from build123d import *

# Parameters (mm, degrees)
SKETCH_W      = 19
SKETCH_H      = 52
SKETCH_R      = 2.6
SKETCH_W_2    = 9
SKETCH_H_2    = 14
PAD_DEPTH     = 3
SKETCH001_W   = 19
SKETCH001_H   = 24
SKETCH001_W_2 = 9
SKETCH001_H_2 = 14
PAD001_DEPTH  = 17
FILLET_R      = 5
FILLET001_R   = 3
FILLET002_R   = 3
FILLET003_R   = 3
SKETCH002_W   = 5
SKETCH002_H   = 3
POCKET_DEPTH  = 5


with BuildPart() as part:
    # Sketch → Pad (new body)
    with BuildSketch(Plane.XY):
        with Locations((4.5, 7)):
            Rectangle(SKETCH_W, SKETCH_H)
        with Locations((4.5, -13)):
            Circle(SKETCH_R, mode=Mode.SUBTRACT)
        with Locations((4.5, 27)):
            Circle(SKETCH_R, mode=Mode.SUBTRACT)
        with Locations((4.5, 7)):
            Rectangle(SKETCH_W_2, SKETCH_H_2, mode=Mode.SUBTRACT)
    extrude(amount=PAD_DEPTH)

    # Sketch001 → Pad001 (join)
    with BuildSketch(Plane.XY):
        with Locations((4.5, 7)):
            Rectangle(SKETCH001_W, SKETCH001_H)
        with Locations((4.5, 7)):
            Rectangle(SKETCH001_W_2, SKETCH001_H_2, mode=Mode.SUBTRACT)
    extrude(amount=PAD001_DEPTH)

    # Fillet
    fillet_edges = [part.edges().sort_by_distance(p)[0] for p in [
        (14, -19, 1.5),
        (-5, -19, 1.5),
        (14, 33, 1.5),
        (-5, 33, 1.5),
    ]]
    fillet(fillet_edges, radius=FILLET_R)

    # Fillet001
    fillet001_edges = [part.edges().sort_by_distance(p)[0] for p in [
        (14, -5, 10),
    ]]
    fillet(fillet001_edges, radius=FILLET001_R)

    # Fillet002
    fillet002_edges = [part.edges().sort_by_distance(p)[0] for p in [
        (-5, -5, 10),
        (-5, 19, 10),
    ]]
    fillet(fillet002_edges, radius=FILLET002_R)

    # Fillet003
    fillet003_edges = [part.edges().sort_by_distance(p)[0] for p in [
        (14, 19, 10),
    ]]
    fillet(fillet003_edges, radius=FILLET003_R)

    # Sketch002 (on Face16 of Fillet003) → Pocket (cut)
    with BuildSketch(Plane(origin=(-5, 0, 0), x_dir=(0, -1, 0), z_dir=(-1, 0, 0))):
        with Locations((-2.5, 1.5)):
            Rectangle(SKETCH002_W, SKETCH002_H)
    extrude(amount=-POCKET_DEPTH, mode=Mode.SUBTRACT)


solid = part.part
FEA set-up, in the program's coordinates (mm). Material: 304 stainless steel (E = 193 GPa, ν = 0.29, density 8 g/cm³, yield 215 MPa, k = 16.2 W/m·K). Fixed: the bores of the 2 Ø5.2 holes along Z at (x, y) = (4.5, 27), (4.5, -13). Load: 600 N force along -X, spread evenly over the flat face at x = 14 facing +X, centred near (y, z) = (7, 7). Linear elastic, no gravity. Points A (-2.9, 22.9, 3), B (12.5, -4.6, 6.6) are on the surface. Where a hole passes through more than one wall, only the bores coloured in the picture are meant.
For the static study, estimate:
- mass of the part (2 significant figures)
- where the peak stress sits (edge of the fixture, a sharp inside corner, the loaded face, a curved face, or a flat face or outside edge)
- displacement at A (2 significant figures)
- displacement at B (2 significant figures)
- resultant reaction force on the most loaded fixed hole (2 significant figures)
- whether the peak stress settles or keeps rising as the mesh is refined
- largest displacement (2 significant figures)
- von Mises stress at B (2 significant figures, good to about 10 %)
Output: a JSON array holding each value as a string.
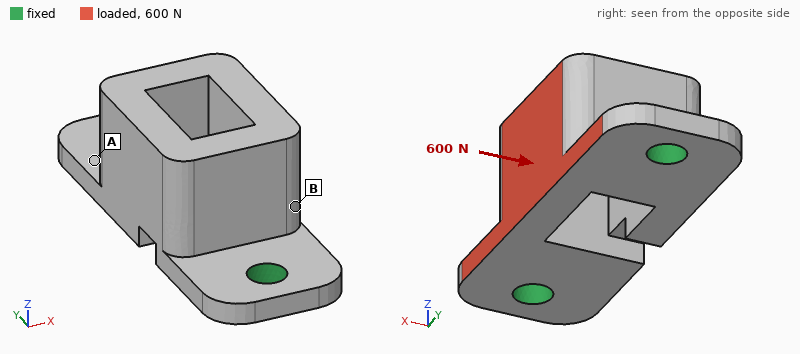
["55 g", "edge of the fixture", "3.4 µm", "7.9 µm", "310 N", "keeps rising", "16 µm", "7.1 MPa"]
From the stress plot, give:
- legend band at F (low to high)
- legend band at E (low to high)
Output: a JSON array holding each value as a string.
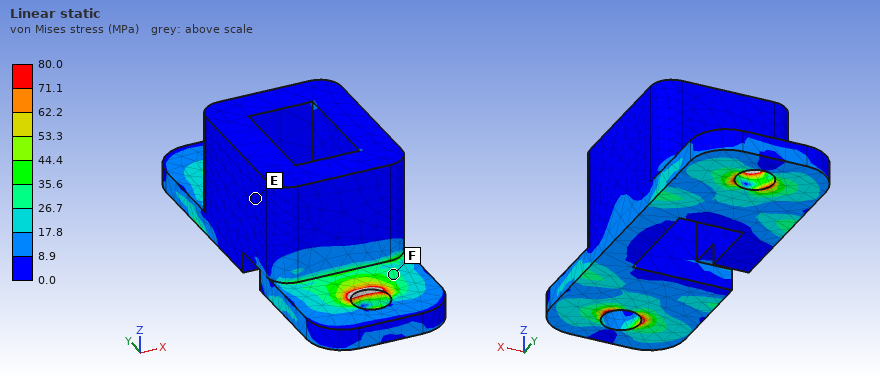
["26.7 to 35.6 MPa", "0.0 to 8.9 MPa"]
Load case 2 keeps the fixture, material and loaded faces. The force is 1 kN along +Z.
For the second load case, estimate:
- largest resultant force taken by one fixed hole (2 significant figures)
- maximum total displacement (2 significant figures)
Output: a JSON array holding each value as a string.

["560 N", "40 µm"]
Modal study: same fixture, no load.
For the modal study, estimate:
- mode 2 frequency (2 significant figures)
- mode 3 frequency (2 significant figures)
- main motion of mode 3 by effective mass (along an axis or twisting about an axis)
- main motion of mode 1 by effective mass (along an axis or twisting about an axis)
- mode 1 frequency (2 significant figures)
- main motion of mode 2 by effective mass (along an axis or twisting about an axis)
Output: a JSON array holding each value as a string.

["10 kHz", "13 kHz", "along Y", "along X", "4700 Hz", "along Z"]
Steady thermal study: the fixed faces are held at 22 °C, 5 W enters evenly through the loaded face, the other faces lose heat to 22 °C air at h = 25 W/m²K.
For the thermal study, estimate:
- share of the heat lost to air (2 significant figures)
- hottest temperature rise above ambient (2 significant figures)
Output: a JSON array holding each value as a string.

["28 %", "33 K"]
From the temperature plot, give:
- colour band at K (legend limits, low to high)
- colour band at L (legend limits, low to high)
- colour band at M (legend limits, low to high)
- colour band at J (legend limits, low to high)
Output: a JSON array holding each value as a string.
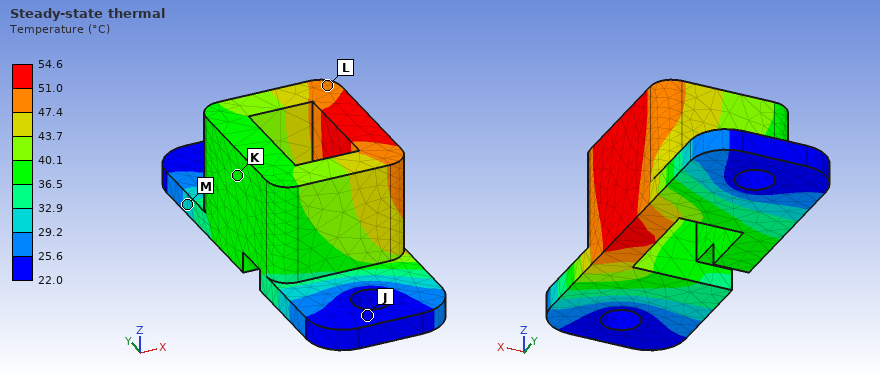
["36.5 to 40.1 °C", "47.4 to 51.0 °C", "29.2 to 32.9 °C", "22.0 to 25.6 °C"]
